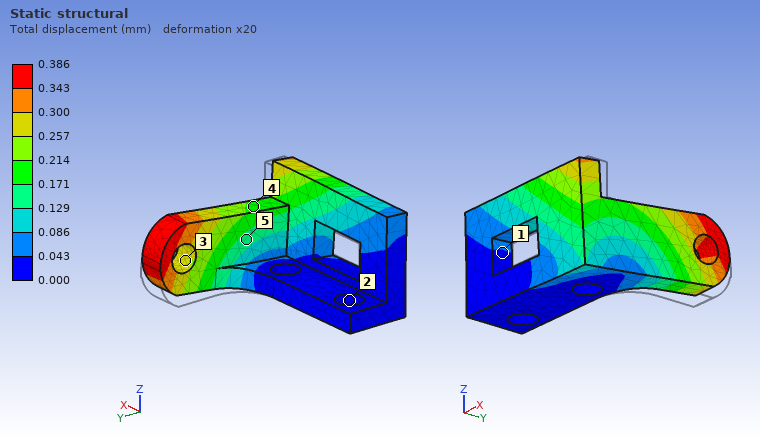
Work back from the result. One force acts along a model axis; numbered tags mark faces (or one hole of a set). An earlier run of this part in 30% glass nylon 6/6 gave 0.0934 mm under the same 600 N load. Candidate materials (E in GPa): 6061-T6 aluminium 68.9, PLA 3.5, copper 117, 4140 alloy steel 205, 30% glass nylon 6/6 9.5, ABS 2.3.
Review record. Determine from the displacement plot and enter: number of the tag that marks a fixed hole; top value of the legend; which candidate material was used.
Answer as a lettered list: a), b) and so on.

a) 2
b) 0.386 mm
c) ABS
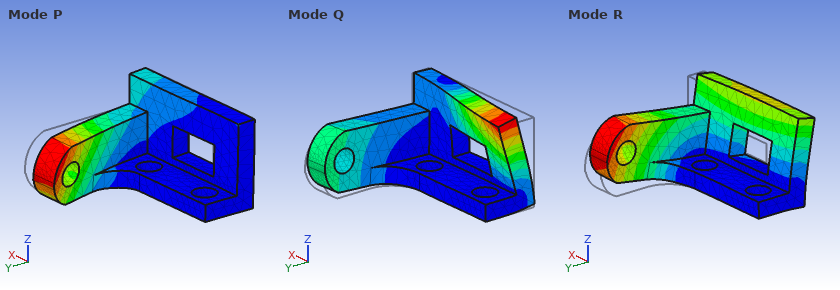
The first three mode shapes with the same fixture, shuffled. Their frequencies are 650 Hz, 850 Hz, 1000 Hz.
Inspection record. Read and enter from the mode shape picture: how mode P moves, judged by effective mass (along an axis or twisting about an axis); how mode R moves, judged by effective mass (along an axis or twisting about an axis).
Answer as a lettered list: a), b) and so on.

a) along X
b) along Y
